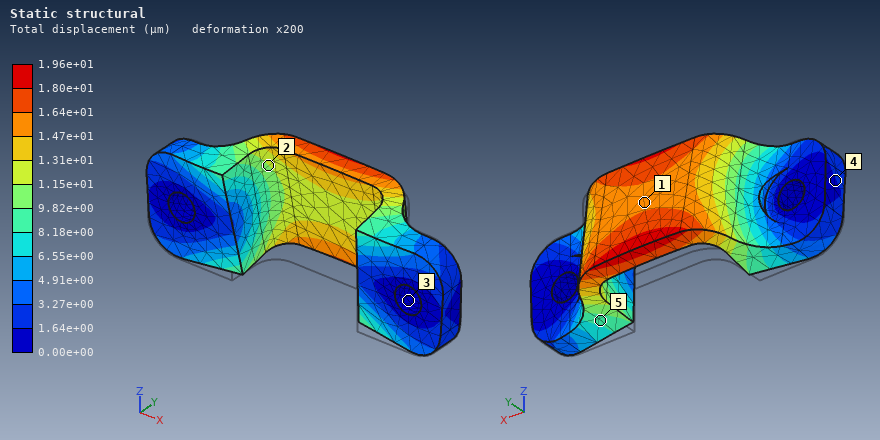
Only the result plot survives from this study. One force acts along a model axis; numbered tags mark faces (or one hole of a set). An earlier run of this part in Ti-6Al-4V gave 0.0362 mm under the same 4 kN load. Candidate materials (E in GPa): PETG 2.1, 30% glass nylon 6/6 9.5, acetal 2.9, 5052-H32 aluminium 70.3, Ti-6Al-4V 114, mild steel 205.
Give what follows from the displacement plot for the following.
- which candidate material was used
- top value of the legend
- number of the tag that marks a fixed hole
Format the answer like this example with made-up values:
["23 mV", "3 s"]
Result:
["mild steel", "1.96e+01 µm", "3"]
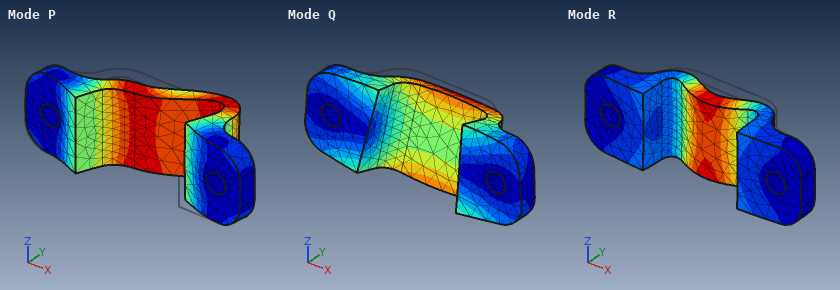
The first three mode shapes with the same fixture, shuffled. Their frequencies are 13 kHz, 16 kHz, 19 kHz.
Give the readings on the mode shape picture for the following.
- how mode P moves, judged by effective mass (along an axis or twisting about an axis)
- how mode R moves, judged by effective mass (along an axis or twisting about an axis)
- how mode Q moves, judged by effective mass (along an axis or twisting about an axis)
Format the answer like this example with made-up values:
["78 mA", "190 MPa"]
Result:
["along X", "along Y", "along Z"]
